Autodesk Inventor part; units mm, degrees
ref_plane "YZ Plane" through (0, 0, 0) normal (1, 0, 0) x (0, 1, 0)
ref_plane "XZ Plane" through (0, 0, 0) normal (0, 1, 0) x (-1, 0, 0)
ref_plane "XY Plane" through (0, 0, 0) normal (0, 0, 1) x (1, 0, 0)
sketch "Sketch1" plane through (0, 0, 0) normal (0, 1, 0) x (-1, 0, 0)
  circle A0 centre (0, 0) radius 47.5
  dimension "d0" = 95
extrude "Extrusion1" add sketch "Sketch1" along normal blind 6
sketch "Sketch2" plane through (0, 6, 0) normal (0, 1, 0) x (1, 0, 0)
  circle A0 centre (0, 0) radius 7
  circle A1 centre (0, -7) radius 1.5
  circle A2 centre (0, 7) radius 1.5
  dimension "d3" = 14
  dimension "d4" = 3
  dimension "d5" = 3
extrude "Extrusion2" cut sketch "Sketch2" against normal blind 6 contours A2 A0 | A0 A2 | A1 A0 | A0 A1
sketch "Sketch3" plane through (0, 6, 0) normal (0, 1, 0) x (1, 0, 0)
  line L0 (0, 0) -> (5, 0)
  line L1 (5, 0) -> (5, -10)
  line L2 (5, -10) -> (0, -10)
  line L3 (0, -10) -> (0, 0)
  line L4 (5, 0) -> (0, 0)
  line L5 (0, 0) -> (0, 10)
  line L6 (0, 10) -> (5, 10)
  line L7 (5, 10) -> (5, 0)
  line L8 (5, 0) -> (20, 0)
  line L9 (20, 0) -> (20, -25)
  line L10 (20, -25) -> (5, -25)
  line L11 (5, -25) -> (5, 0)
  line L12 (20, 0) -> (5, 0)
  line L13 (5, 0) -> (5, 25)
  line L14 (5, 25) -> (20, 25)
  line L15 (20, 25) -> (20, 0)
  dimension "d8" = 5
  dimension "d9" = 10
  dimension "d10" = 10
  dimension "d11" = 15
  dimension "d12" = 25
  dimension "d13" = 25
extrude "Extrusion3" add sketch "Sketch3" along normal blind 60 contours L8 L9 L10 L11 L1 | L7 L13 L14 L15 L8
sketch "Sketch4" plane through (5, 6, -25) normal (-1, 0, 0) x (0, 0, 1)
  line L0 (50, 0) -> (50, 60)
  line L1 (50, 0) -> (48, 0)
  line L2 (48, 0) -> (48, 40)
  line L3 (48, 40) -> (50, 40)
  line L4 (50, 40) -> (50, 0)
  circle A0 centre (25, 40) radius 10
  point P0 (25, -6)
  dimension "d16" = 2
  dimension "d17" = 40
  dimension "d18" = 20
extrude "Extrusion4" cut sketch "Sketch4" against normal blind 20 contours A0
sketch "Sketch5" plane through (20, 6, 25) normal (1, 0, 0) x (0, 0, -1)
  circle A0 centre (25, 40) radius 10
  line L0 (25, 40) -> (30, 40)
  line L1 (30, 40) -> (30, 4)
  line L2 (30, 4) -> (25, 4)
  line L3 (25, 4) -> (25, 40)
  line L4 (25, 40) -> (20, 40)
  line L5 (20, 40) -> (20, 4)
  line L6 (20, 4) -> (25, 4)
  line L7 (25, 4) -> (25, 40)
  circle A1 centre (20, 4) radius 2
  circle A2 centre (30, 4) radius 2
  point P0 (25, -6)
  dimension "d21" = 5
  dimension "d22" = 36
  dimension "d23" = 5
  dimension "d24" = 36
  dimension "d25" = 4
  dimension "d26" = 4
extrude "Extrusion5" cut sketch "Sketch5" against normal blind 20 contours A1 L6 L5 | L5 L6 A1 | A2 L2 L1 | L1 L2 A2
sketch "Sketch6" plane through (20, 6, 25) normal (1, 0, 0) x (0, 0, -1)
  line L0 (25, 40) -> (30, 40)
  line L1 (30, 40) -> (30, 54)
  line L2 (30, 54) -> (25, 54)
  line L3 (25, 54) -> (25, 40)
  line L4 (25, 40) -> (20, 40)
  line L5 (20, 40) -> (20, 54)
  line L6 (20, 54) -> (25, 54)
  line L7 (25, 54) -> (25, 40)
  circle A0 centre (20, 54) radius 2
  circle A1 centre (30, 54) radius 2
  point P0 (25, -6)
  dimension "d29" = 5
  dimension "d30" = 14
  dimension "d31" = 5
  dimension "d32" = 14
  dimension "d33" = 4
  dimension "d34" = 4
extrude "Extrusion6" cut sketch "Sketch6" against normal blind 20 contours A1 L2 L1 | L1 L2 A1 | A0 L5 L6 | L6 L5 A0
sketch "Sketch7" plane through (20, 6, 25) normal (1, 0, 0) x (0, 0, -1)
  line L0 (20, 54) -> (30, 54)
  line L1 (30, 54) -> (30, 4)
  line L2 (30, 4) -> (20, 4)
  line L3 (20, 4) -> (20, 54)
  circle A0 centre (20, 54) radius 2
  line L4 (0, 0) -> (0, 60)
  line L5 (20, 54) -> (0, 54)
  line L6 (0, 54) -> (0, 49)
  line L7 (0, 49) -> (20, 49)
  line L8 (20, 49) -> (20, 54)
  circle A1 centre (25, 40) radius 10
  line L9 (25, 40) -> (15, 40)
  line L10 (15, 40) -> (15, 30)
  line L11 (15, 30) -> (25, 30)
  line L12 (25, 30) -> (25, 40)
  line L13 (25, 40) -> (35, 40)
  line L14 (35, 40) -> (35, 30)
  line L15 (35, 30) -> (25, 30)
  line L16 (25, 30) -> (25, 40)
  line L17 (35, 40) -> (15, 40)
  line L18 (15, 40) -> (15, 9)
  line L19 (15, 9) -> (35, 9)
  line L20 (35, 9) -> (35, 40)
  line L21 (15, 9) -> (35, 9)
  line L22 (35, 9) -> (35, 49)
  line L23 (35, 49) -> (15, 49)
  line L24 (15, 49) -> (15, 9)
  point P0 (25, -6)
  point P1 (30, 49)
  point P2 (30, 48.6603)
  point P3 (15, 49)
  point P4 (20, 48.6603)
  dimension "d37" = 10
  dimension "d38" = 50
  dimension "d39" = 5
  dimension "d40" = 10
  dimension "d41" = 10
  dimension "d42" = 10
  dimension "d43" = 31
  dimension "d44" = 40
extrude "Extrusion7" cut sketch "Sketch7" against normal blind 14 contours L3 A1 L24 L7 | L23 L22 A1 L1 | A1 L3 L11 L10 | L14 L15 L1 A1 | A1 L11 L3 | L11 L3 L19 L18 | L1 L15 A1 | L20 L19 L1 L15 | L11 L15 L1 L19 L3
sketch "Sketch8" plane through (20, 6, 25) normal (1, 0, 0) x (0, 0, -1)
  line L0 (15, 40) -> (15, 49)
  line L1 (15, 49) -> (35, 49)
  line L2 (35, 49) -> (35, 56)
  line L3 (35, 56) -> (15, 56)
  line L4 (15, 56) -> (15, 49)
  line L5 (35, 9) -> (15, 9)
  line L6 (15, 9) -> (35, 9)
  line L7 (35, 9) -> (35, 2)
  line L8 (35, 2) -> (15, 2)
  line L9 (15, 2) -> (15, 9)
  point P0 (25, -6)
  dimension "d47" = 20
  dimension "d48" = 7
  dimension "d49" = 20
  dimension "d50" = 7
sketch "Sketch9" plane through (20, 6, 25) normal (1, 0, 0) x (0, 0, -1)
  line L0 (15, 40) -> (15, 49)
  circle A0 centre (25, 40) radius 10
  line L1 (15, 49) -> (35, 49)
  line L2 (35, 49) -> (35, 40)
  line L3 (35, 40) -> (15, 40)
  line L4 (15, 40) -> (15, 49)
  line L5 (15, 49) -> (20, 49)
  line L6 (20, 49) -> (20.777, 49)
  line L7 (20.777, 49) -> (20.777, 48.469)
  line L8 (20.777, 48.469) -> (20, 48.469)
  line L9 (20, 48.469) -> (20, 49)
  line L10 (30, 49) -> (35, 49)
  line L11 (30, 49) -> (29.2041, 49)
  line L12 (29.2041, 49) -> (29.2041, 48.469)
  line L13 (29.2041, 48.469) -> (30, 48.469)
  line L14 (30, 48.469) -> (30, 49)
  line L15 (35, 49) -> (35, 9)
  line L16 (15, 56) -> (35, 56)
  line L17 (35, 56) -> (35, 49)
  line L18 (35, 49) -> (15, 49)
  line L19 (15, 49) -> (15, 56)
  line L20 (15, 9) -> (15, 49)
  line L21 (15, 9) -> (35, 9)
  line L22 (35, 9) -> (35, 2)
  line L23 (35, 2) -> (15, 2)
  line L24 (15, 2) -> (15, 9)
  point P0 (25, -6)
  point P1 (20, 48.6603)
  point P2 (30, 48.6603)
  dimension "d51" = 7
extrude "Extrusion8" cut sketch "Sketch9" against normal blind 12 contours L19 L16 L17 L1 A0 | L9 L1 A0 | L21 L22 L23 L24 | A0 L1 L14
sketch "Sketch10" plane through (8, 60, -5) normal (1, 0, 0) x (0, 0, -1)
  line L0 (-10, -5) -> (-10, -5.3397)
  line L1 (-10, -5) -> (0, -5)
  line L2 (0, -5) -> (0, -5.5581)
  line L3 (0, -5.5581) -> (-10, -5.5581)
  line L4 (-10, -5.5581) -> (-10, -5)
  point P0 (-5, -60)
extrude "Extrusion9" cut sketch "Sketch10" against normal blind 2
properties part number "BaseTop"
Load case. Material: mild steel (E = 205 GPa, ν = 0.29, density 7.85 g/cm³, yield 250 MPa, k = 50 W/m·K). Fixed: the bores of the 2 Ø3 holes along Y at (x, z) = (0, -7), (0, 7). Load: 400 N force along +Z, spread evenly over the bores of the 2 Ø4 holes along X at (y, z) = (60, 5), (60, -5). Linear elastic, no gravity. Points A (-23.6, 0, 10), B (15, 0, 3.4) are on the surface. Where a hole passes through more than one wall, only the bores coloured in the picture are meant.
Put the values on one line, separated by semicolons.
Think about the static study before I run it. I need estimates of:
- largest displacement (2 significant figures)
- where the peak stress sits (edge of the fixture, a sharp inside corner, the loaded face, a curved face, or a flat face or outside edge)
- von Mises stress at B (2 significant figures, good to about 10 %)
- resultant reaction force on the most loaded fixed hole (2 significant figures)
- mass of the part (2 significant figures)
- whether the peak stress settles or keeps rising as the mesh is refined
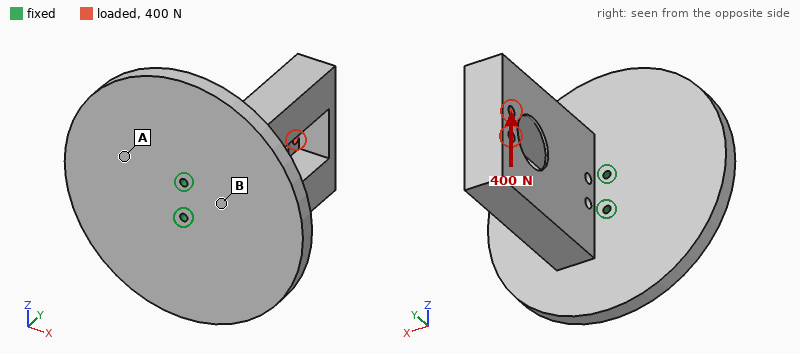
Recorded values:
29 µm; edge of the fixture; 8.6 MPa; 1.1 kN; 570 g; keeps rising
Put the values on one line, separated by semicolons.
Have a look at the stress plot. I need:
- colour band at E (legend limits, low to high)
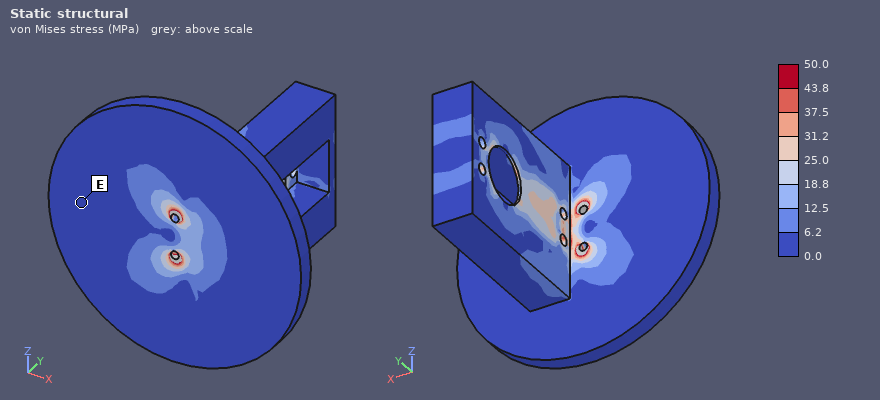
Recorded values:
0.0 to 6.2 MPa
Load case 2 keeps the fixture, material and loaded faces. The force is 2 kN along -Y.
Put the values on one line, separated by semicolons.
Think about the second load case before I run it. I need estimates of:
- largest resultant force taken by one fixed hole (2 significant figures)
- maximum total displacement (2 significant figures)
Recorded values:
1.0 kN; 22 µm
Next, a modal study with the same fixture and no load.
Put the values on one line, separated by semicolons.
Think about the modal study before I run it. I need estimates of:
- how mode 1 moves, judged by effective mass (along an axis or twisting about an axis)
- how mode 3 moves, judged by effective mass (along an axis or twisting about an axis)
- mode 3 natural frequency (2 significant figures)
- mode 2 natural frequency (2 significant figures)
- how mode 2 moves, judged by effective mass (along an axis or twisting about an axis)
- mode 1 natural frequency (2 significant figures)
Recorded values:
along X; along Y; 2400 Hz; 1700 Hz; along Z; 950 Hz
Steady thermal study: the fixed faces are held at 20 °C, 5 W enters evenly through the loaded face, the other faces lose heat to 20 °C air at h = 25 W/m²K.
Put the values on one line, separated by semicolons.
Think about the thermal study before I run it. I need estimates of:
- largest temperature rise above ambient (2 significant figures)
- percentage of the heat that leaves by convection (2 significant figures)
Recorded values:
21 K; 49 %
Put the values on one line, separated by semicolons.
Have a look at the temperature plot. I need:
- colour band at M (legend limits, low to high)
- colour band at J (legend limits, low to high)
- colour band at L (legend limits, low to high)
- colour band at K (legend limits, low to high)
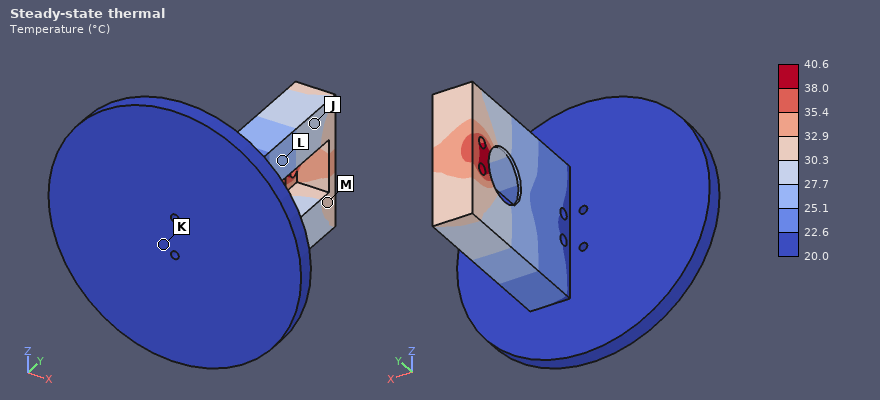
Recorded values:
30.3 to 32.9 °C; 27.7 to 30.3 °C; 25.1 to 27.7 °C; 20.0 to 22.6 °C
